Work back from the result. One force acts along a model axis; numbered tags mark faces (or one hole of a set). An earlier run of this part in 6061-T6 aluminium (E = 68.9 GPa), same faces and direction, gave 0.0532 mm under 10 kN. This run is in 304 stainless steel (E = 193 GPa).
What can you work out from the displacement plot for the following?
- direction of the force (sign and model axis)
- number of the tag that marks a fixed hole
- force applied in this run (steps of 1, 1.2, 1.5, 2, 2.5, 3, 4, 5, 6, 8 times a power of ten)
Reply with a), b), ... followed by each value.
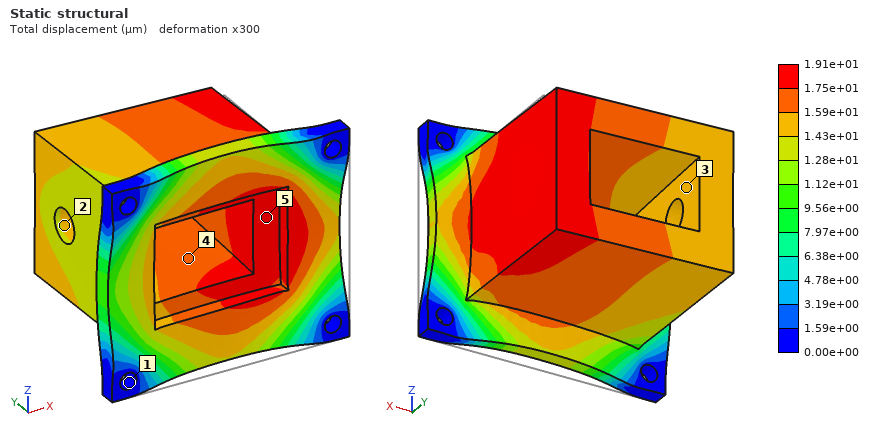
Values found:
a) +Y
b) 1
c) 10 kN
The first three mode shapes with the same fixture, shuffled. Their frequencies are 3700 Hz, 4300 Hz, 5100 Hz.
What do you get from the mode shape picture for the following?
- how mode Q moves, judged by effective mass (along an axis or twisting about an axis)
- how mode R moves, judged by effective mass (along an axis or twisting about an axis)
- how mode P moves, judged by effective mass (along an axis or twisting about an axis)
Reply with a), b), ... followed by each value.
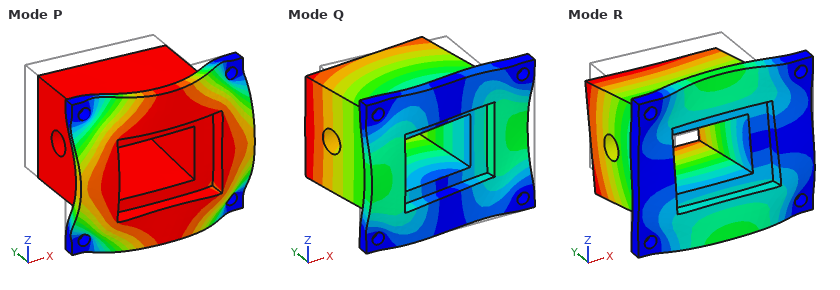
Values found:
a) along X
b) along Z
c) along Y
